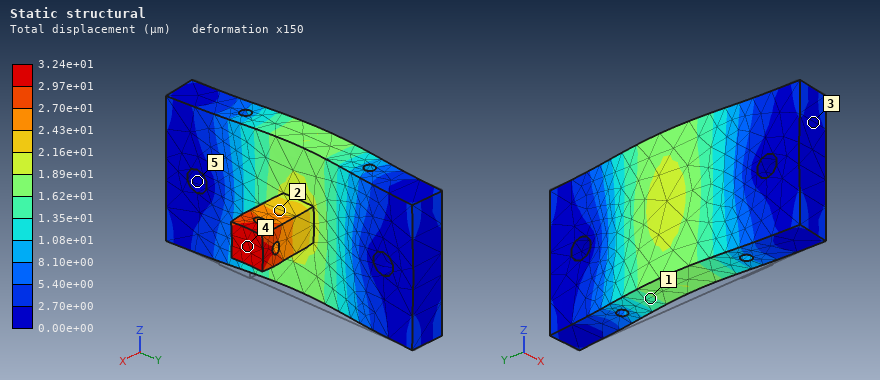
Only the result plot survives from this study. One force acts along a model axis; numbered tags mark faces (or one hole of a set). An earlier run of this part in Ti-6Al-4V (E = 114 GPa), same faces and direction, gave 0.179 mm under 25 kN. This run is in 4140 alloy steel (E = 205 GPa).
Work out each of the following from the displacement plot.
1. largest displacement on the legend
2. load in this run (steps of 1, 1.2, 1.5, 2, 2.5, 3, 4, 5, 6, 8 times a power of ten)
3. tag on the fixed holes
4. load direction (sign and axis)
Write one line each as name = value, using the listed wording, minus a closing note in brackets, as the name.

largest displacement on the legend = 3.24e+01 µm
load in this run = 8 kN
tag on the fixed holes = 5
load direction = -X
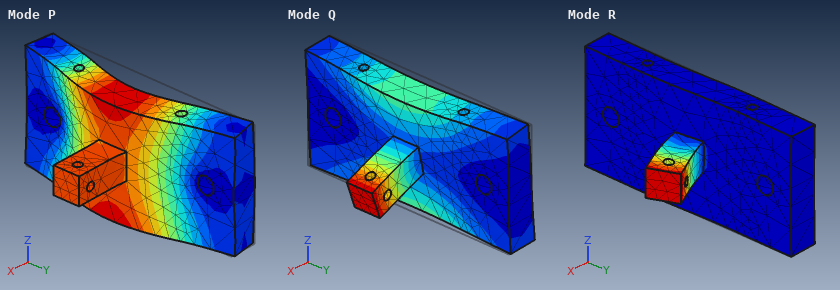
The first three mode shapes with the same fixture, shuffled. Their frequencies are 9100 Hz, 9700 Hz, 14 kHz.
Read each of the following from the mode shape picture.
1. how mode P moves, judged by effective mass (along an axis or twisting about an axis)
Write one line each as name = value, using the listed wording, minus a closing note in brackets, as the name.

how mode P moves, judged by effective mass = along X
